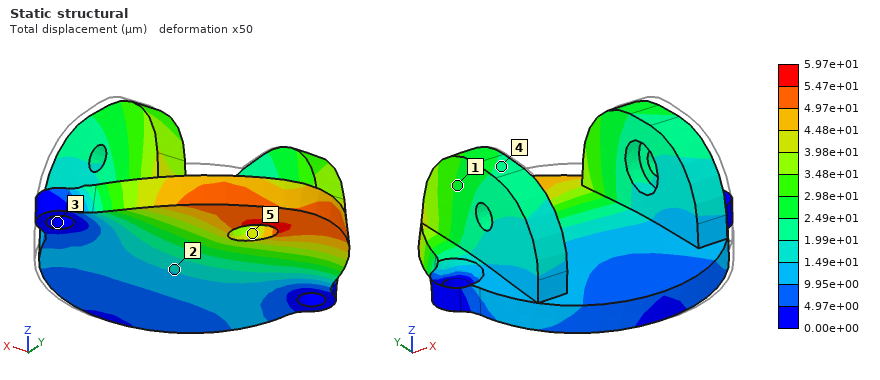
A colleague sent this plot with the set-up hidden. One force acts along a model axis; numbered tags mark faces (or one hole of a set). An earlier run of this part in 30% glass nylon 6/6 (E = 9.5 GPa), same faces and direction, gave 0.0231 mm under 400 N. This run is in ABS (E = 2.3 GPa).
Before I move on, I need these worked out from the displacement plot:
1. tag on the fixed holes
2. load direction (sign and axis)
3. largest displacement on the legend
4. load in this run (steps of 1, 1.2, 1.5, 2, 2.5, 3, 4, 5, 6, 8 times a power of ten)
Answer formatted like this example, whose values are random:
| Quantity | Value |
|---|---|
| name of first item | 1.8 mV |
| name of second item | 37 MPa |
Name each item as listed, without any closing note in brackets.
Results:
| Quantity | Value |
|---|---|
| tag on the fixed holes | 3 |
| load direction | -X |
| largest displacement on the legend | 5.97e+01 µm |
| load in this run | 250 N |
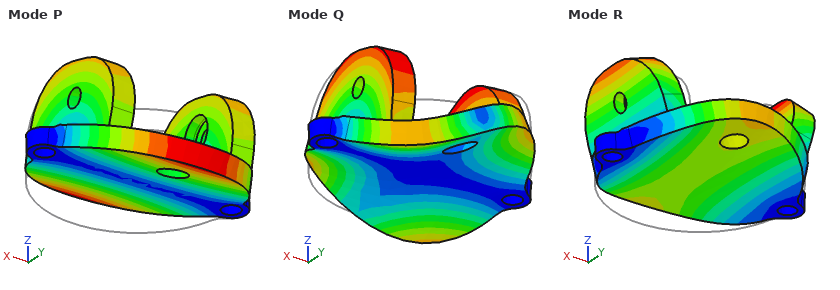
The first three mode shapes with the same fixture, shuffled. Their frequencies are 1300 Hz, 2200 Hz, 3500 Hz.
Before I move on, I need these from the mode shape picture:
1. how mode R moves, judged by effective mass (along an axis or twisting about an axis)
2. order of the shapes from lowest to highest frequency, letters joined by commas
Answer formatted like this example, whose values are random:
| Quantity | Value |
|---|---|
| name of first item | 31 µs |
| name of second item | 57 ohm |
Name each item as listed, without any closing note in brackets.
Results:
| Quantity | Value |
|---|---|
| how mode R moves, judged by effective mass | along Z |
| order of the shapes from lowest to highest frequency, letters joined by commas | P, R, Q |
